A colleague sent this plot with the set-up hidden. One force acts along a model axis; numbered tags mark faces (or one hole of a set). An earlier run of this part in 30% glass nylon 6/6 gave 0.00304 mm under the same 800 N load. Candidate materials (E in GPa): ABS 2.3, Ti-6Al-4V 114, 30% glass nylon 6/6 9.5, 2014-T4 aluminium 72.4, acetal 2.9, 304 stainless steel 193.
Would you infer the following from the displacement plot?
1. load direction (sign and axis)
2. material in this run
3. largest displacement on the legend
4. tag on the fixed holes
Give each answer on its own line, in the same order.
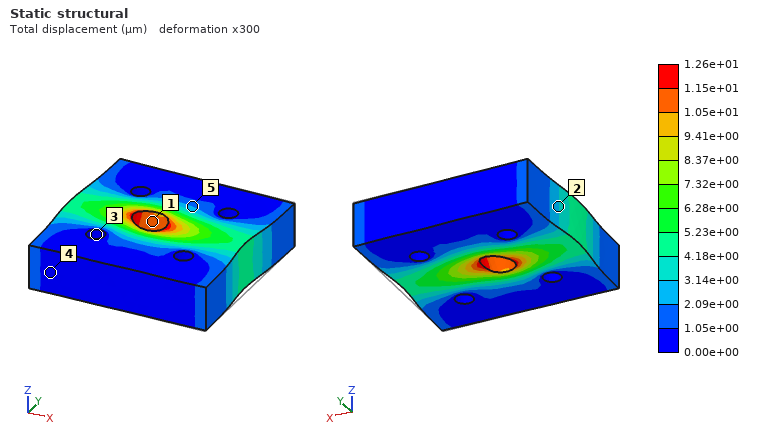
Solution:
-X
ABS
1.26e+01 µm
3
